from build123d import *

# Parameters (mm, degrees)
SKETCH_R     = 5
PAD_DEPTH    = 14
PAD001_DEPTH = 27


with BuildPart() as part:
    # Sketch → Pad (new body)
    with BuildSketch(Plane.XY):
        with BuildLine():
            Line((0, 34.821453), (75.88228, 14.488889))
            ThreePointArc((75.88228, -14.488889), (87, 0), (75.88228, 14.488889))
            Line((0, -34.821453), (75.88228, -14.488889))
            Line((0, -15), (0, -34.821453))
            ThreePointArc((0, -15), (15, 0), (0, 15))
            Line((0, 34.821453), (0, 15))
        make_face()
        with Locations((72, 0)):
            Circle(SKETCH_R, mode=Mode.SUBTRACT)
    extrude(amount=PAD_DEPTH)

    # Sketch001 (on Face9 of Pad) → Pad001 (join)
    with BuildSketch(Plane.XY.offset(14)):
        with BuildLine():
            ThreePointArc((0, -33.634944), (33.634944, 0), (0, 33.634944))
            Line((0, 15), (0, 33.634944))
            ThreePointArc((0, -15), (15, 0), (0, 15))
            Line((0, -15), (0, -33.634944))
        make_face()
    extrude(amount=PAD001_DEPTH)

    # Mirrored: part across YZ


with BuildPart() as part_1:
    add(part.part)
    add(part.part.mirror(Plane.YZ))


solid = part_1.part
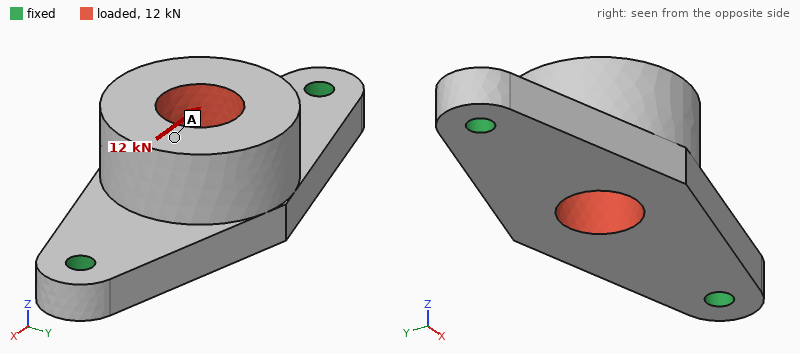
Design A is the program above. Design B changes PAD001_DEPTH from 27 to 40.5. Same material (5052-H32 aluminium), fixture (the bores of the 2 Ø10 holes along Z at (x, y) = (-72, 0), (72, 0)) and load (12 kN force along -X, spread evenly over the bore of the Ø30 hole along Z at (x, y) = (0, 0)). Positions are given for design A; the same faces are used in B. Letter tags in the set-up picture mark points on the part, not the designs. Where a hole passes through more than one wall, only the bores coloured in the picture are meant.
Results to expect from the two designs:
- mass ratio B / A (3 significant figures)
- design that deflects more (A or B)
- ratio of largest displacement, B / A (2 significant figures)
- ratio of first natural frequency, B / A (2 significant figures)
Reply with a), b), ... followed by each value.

a) 1.22
b) B
c) 1.7
d) 0.72
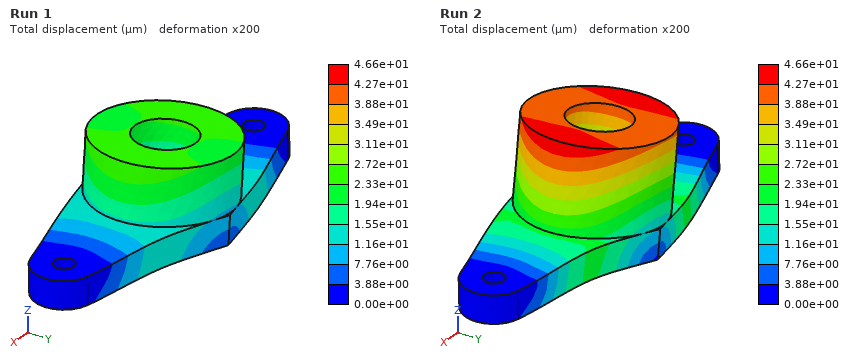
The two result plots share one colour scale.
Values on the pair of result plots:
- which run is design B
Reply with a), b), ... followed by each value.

a) Run 2
